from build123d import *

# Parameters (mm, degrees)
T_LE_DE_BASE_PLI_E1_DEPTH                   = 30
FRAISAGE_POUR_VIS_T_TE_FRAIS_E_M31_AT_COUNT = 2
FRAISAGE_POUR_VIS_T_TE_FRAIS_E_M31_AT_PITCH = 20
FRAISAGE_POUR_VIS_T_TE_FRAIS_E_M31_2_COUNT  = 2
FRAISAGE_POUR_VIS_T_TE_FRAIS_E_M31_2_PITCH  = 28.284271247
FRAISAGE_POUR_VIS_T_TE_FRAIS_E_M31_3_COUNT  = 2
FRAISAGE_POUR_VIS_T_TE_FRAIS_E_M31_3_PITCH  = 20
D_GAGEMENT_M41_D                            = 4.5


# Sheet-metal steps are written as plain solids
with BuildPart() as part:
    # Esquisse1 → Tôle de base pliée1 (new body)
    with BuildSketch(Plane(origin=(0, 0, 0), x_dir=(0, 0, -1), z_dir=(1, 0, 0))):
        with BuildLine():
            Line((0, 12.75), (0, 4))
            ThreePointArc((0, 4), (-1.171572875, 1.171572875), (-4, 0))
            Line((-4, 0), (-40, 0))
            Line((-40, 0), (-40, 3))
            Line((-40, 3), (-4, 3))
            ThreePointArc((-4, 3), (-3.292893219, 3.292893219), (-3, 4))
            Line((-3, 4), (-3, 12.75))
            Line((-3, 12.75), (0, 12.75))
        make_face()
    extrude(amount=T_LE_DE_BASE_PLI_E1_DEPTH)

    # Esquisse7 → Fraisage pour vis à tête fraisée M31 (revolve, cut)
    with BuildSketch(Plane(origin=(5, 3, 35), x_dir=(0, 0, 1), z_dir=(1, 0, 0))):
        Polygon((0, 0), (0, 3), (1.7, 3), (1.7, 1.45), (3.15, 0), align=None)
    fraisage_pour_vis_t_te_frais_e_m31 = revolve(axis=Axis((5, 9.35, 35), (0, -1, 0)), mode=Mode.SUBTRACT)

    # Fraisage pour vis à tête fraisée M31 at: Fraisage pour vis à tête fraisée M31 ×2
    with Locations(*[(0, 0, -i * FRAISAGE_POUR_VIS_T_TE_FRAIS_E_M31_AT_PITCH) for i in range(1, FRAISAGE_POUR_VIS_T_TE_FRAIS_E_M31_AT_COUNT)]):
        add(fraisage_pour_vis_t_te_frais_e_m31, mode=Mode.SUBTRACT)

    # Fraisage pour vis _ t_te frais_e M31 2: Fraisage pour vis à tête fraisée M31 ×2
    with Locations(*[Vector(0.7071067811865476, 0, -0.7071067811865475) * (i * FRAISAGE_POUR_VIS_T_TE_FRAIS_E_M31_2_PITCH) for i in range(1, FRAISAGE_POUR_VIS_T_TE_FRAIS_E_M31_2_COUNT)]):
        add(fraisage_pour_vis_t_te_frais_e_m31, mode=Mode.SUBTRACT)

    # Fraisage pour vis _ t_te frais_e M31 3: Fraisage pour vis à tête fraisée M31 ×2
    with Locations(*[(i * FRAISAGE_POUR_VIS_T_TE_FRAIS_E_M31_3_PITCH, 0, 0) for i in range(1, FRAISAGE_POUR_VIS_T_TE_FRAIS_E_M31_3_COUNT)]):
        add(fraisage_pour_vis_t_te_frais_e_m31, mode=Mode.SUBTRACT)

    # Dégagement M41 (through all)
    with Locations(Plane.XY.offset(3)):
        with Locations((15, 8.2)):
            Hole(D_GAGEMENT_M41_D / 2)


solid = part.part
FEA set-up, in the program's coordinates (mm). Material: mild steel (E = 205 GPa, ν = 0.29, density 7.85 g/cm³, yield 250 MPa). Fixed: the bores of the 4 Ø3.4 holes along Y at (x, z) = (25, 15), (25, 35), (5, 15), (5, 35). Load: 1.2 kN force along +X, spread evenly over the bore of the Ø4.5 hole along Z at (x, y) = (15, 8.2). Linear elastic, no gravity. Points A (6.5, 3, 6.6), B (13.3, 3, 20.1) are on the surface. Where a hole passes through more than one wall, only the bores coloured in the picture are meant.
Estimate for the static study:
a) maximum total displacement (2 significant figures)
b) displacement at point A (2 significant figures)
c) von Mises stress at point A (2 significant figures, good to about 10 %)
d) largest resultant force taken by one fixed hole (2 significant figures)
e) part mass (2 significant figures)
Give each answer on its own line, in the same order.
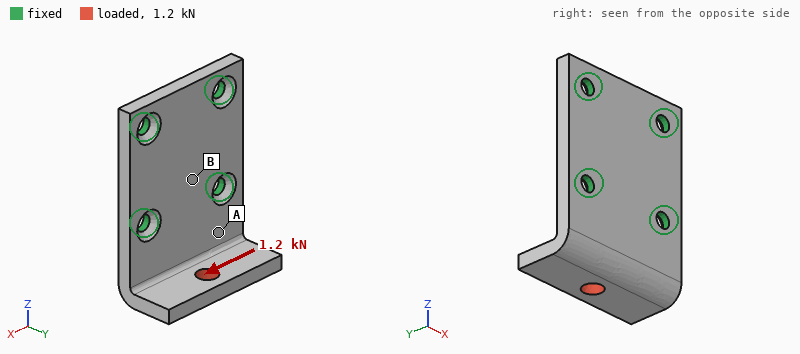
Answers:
48 µm
12 µm
110 MPa
1.0 kN
33 g
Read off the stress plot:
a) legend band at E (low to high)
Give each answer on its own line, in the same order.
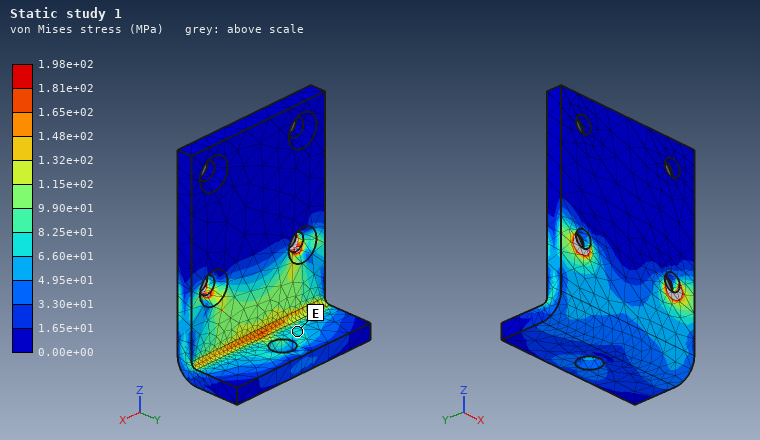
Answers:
6.60e+01 to 8.25e+01 MPa
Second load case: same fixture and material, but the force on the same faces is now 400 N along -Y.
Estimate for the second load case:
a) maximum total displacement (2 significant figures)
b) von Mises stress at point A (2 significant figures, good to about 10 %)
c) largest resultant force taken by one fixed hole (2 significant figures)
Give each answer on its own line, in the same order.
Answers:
54 µm
38 MPa
310 N
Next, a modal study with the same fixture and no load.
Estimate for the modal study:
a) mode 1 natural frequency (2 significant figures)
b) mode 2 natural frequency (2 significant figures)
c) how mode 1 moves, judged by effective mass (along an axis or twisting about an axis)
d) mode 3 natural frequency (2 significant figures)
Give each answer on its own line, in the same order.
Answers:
4800 Hz
8500 Hz
along Y
16 kHz
